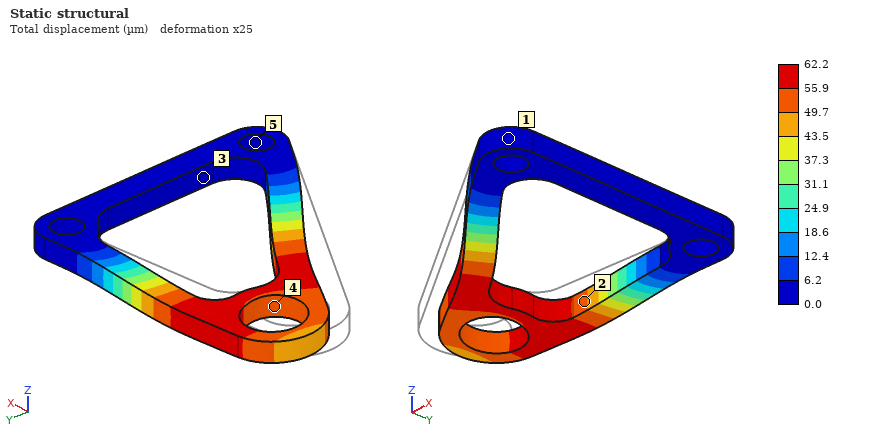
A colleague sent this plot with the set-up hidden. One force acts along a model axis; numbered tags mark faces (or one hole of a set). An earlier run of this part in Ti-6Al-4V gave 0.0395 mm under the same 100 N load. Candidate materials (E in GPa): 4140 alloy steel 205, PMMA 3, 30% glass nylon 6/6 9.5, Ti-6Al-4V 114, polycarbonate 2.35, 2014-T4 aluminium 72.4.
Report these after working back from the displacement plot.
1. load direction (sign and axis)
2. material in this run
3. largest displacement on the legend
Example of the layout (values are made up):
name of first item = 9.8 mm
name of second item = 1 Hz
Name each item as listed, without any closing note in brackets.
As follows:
load direction = +Y
material in this run = 2014-T4 aluminium
largest displacement on the legend = 62.2 µm
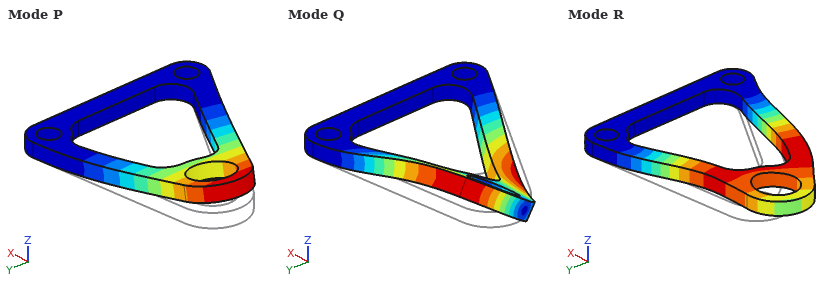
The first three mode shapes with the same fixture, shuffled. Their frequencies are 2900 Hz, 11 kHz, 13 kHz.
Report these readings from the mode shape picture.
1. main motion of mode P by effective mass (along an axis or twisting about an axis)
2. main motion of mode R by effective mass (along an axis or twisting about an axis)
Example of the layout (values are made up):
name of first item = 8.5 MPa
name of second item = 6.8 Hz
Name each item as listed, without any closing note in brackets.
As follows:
main motion of mode P by effective mass = along Z
main motion of mode R by effective mass = along Y
